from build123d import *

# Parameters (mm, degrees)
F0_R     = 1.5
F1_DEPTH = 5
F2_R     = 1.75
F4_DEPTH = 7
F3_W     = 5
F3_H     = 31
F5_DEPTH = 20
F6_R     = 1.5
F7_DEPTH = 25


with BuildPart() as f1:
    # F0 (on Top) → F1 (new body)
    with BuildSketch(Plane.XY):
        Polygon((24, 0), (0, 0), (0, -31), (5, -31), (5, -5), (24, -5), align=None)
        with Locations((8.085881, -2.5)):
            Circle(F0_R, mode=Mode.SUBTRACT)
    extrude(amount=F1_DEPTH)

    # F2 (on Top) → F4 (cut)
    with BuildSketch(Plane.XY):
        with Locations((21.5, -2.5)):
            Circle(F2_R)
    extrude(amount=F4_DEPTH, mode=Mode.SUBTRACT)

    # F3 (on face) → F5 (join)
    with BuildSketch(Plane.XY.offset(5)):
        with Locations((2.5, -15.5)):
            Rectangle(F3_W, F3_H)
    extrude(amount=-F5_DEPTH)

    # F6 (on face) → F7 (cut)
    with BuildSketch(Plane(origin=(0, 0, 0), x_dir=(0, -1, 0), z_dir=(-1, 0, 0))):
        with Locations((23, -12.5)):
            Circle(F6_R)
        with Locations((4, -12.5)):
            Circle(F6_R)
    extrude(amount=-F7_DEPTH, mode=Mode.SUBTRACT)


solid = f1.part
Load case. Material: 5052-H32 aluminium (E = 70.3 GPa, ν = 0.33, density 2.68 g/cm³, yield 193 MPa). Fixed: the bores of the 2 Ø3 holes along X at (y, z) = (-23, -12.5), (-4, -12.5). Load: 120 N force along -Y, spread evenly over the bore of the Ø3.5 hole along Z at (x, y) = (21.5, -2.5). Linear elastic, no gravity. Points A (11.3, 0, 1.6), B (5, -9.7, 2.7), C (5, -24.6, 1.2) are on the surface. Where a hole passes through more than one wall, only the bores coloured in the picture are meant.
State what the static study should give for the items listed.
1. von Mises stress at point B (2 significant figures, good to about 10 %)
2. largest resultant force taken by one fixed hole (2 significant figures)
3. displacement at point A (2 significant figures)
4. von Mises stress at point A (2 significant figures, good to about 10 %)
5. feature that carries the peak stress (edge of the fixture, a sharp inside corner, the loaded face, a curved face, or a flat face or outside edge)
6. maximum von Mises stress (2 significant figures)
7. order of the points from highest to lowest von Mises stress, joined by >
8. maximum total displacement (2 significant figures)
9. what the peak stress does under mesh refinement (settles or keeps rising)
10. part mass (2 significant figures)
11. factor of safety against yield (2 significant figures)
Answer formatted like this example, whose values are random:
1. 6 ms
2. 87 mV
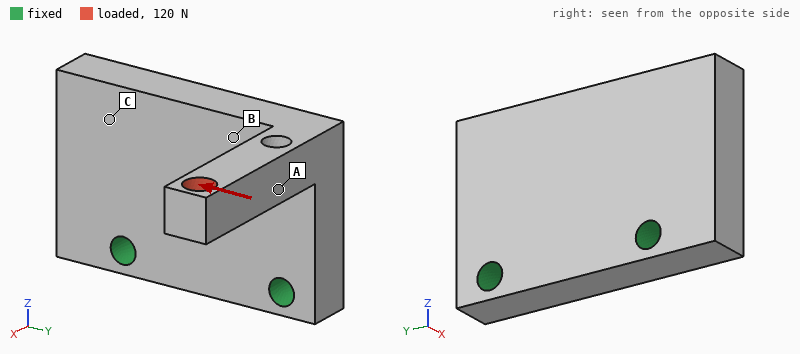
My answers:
1. 29 MPa
2. 150 N
3. 0.049 mm
4. 59 MPa
5. a flat face or outside edge
6. 170 MPa
7. A > B > C
8. 0.15 mm
9. settles
10. 9.2 g
11. 1.1
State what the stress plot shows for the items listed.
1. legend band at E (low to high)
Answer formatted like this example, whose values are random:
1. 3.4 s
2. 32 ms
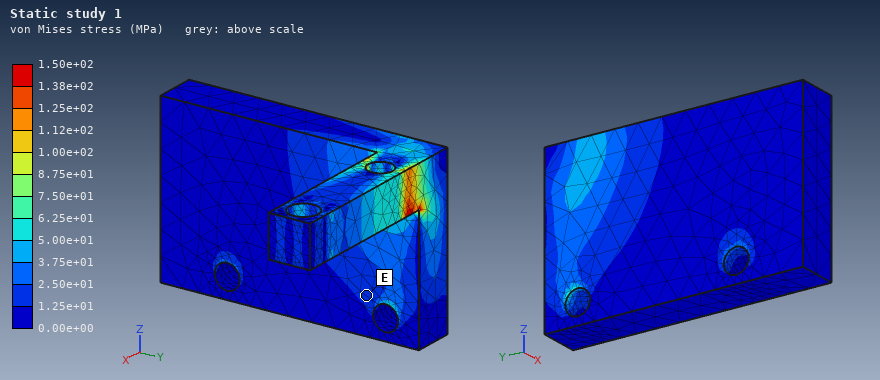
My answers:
1. 1.25e+01 to 2.50e+01 MPa
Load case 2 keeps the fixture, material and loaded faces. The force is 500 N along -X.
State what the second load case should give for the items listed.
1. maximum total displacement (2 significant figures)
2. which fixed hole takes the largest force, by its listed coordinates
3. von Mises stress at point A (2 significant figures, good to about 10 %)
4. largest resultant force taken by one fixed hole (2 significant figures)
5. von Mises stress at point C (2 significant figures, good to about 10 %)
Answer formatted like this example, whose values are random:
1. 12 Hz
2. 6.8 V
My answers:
1. 0.14 mm
2. (-4, -12.5)
3. 33 MPa
4. 500 N
5. 15 MPa
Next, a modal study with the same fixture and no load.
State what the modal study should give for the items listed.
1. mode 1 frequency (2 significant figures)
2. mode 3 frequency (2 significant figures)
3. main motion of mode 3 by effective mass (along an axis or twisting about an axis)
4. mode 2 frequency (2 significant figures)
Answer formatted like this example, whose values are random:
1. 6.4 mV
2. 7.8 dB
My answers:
1. 6200 Hz
2. 11 kHz
3. along X
4. 7600 Hz
